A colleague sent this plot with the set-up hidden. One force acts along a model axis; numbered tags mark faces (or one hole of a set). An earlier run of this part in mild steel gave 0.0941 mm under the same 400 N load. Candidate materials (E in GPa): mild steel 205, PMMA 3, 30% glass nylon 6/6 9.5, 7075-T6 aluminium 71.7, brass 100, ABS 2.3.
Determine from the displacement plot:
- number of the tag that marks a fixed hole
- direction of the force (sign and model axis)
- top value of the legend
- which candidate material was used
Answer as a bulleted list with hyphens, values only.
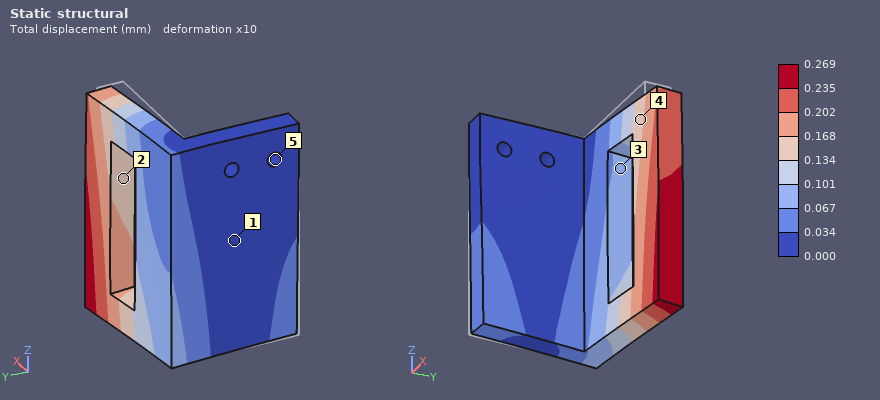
- 5
- +Y
- 0.269 mm
- 7075-T6 aluminium
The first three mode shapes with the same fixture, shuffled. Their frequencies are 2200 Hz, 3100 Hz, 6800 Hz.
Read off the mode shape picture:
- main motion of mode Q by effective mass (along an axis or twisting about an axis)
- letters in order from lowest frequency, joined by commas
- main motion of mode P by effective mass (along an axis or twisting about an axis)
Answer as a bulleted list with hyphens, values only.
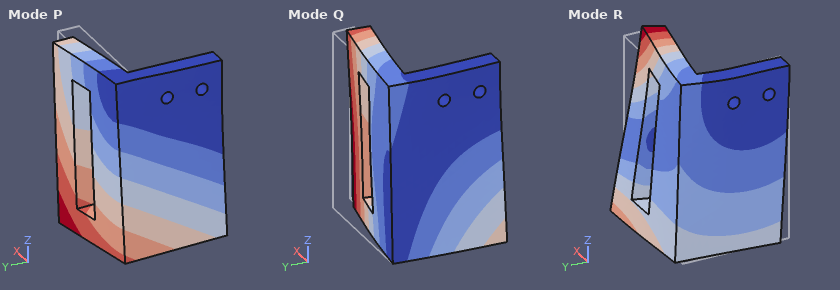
- along Y
- P, Q, R
- along X
